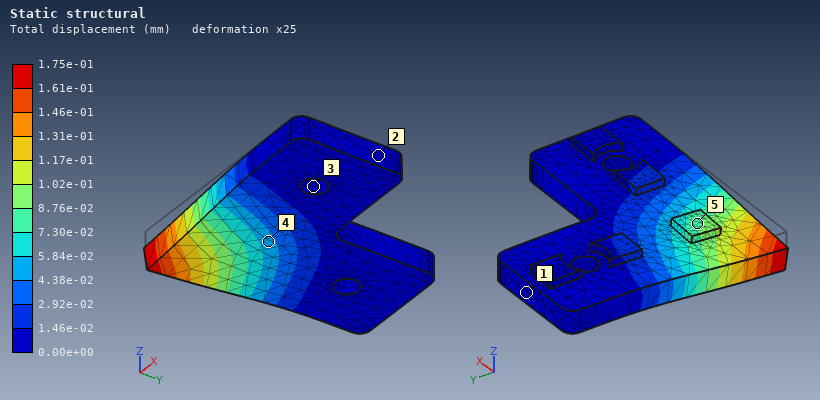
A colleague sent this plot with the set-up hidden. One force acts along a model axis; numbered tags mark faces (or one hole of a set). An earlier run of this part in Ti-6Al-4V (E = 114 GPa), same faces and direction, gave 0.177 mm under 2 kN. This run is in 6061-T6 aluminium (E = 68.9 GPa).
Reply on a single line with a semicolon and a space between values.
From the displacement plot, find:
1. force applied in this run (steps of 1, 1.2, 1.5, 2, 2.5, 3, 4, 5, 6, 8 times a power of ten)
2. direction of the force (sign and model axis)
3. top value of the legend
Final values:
1.2 kN; -Z; 1.75e-01 mm
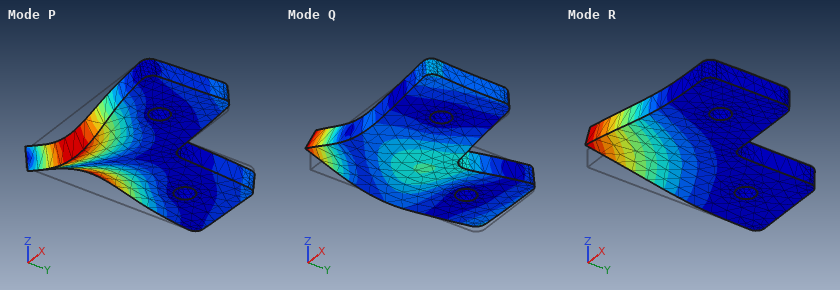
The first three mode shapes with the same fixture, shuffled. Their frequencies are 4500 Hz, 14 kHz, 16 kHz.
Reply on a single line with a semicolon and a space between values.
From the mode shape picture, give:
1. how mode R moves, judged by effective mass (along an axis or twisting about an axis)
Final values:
along Z
